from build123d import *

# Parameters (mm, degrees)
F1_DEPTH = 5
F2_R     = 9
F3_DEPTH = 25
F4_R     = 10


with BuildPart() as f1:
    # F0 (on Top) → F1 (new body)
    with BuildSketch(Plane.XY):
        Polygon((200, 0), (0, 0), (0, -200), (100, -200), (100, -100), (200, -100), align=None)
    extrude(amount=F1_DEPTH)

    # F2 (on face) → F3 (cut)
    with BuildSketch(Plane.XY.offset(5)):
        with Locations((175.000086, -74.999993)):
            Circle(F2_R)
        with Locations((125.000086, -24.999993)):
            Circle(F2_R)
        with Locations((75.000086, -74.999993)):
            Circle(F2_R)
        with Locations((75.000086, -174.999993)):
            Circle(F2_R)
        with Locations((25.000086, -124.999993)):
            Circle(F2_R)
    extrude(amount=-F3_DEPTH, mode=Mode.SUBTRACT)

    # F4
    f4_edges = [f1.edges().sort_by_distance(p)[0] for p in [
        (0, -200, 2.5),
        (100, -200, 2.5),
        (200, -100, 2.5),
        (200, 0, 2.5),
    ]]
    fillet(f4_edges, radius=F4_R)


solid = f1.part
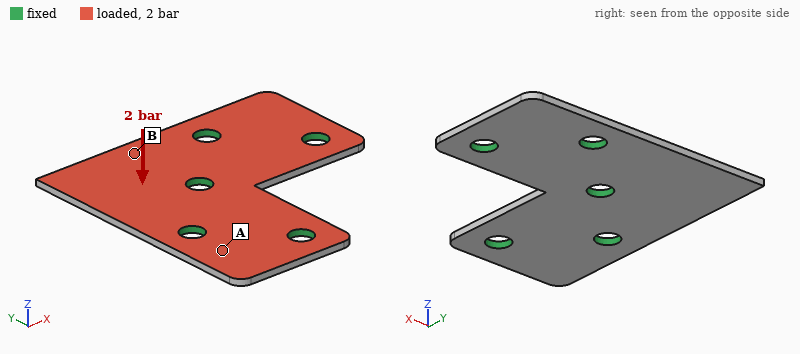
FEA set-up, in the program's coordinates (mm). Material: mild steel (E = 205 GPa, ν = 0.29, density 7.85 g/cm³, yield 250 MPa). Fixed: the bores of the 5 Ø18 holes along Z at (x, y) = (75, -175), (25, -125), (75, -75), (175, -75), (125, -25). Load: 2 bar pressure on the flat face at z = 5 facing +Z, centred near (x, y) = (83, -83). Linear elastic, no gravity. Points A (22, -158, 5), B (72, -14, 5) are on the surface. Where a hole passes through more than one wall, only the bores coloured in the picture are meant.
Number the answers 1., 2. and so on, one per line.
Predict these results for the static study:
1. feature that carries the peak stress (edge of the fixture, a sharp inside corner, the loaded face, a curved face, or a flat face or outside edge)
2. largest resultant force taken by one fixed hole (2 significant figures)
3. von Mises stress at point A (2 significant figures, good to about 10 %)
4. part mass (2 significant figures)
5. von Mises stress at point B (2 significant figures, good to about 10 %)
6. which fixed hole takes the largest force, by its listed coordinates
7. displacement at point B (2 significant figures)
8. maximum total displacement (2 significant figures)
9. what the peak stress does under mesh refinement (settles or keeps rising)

1. edge of the fixture
2. 1.8 kN
3. 17 MPa
4. 1.1 kg
5. 42 MPa
6. (75, -75)
7. 0.12 mm
8. 0.51 mm
9. keeps rising
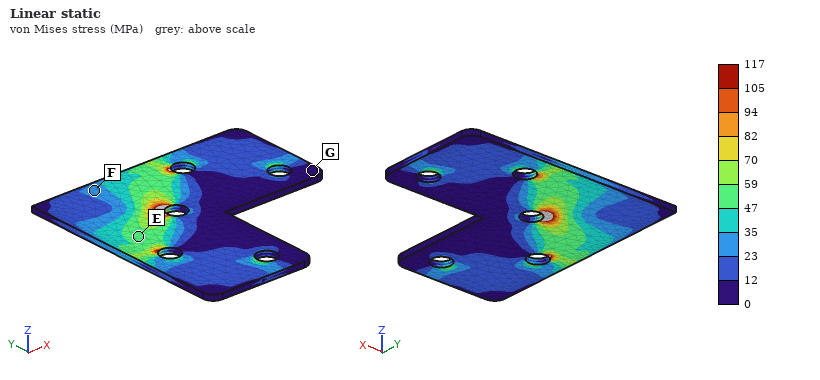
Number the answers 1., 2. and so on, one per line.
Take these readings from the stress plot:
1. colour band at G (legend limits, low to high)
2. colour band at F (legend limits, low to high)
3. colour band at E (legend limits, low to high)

1. 0 to 12 MPa
2. 23 to 35 MPa
3. 47 to 59 MPa
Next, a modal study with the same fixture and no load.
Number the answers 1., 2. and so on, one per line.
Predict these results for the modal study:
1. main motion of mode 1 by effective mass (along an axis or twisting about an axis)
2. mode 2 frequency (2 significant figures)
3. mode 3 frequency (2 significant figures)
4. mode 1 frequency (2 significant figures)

1. along Z
2. 1700 Hz
3. 1700 Hz
4. 730 Hz
